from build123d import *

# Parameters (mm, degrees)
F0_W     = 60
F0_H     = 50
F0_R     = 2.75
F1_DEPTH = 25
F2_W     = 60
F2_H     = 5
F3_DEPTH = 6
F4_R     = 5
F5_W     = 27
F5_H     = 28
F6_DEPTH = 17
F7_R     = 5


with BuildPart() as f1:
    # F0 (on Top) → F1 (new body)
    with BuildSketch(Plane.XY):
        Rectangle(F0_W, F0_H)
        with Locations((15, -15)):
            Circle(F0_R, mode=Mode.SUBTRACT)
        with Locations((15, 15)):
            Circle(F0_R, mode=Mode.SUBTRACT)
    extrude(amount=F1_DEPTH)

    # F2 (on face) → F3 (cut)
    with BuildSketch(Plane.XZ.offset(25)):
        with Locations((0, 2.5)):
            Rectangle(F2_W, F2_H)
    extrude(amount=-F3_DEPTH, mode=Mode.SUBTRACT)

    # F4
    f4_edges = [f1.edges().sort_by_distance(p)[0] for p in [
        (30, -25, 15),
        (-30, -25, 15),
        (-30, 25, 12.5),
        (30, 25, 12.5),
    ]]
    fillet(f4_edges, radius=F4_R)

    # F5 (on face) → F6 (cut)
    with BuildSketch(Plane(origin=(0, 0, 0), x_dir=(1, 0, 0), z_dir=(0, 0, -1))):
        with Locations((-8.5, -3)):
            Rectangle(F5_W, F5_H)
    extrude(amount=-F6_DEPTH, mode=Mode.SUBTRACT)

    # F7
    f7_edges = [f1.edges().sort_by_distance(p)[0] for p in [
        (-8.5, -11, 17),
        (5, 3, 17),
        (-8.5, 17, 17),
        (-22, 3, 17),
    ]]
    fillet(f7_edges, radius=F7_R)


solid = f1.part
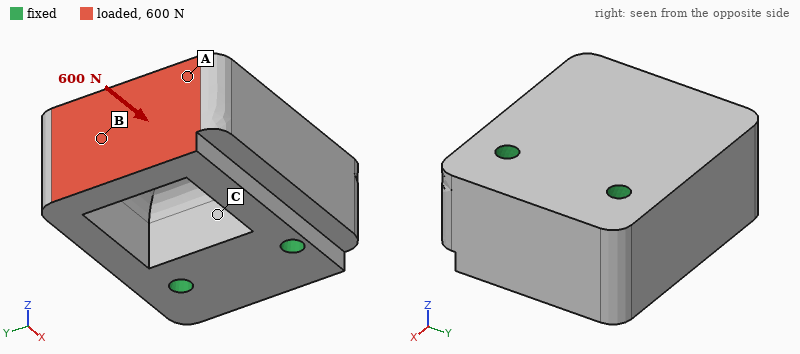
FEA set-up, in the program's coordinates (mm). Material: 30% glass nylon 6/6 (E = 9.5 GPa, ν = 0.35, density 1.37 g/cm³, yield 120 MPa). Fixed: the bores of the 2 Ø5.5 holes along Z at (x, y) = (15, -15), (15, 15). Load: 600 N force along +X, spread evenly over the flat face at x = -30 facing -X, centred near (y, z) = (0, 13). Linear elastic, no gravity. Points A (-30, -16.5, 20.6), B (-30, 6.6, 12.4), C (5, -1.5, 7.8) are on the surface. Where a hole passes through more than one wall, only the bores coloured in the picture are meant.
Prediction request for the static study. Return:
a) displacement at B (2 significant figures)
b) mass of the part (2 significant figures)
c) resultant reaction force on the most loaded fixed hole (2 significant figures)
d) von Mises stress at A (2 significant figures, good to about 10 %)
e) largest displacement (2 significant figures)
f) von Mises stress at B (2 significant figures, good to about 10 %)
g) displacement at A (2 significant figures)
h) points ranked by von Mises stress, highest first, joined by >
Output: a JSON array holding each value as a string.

["11 µm", "81 g", "310 N", "0.73 MPa", "19 µm", "1.4 MPa", "6.0 µm", "B > A > C"]
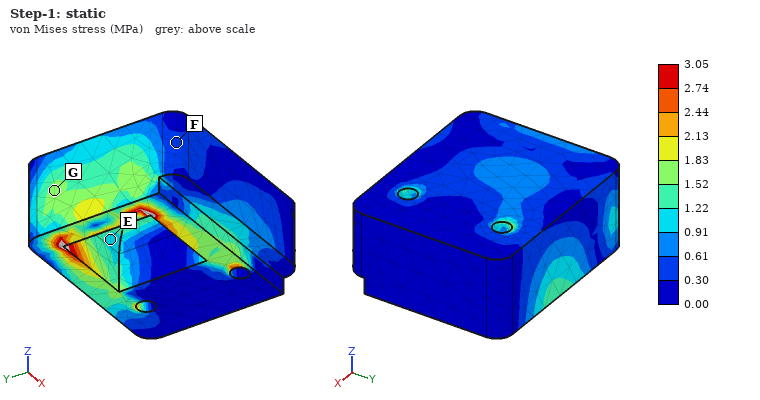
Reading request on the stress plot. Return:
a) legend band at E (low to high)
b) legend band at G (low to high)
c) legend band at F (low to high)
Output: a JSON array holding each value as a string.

["0.91 to 1.22 MPa", "1.52 to 1.83 MPa", "0.30 to 0.61 MPa"]
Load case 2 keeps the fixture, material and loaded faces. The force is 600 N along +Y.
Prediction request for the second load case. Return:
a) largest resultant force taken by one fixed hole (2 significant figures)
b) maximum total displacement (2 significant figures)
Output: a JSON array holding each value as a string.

["840 N", "50 µm"]
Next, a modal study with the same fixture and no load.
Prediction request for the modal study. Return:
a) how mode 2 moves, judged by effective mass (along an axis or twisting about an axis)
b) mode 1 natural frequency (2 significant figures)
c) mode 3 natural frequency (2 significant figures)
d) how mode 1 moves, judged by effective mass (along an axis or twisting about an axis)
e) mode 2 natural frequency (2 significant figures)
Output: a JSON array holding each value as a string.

["along Y", "3600 Hz", "6500 Hz", "along Z", "4200 Hz"]
